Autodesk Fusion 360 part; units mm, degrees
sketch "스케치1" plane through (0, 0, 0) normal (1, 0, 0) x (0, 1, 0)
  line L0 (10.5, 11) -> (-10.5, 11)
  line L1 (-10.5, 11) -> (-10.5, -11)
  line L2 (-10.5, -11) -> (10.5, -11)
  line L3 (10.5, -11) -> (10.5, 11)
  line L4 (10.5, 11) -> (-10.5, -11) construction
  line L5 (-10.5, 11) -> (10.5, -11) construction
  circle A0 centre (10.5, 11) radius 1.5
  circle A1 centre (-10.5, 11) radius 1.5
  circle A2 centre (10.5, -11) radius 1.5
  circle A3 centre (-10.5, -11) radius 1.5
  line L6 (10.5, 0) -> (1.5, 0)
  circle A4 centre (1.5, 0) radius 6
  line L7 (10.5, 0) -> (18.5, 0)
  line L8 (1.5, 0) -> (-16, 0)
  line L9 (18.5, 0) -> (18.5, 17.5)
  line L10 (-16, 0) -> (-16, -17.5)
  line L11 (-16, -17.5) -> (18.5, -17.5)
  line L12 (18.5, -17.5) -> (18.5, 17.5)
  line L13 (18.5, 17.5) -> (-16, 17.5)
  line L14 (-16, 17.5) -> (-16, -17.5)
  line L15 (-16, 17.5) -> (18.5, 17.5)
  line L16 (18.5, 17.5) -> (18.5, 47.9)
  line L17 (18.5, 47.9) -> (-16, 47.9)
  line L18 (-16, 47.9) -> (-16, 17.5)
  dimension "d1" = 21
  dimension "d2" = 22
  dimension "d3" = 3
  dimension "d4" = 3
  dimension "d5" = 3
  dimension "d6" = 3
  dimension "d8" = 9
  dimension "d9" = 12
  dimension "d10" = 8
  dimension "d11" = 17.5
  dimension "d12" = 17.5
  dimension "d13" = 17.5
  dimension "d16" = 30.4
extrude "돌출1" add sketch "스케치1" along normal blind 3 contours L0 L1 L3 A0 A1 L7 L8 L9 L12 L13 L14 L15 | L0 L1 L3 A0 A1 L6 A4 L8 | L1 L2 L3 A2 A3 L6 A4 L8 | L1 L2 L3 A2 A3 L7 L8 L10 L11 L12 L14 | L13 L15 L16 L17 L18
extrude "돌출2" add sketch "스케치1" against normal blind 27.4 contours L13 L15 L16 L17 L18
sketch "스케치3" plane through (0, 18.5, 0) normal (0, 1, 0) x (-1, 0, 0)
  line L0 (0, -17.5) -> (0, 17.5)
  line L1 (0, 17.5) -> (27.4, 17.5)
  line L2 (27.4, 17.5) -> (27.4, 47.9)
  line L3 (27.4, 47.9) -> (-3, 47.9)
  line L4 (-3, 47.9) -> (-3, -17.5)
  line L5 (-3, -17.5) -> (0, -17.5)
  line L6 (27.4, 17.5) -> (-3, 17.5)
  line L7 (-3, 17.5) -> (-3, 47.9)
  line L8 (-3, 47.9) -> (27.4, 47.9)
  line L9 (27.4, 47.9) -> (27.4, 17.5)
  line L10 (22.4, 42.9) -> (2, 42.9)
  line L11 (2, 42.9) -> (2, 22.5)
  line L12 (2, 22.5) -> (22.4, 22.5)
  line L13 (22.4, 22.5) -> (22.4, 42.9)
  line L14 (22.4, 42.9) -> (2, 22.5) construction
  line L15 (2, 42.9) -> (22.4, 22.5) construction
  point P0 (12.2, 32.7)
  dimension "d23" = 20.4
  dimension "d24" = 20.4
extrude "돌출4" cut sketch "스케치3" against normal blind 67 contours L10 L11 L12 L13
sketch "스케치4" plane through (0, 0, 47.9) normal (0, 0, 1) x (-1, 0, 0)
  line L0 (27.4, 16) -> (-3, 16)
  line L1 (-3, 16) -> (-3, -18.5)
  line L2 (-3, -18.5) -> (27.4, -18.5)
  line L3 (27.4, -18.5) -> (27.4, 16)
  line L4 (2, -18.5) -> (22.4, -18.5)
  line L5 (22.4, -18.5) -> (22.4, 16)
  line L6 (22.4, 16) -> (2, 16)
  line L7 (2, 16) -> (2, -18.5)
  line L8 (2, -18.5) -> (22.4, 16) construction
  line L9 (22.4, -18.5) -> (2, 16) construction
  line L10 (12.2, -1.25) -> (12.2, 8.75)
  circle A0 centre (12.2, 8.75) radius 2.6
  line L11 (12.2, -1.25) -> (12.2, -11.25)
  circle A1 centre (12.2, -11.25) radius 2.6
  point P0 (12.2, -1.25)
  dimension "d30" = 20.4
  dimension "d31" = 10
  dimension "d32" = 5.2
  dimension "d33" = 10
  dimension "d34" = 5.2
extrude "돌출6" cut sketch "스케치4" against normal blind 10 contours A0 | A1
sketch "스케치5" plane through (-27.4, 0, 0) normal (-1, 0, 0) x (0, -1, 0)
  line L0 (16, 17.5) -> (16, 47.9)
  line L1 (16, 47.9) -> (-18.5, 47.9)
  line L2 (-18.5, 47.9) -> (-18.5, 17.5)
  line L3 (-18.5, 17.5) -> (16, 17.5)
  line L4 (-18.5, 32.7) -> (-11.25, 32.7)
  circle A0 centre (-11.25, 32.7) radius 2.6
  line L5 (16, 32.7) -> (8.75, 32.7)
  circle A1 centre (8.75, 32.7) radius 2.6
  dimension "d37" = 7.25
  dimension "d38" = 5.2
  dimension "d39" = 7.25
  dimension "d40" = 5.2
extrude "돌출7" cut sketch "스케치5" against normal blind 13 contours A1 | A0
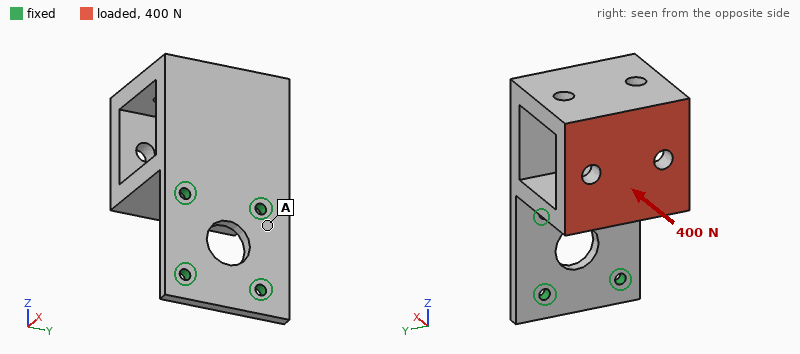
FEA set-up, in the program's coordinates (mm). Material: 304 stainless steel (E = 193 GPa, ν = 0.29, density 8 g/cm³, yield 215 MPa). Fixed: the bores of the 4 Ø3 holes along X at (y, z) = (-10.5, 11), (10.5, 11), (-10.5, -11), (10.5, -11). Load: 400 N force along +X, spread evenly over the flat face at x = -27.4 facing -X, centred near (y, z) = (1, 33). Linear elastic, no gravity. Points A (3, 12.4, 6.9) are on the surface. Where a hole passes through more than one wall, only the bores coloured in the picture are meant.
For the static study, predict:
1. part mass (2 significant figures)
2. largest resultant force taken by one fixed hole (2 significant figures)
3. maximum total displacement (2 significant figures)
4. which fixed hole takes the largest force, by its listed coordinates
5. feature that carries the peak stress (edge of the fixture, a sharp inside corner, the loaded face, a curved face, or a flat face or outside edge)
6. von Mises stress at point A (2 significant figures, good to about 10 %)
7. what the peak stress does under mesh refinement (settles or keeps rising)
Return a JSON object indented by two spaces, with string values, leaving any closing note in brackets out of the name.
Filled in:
{
  "part mass": "160 g",
  "largest resultant force taken by one fixed hole": "260 N",
  "maximum total displacement": "0.18 mm",
  "which fixed hole takes the largest force, by its listed coordinates": "(10.5, 11)",
  "feature that carries the peak stress": "edge of the fixture",
  "von Mises stress at point A": "20 MPa",
  "what the peak stress does under mesh refinement": "keeps rising"
}
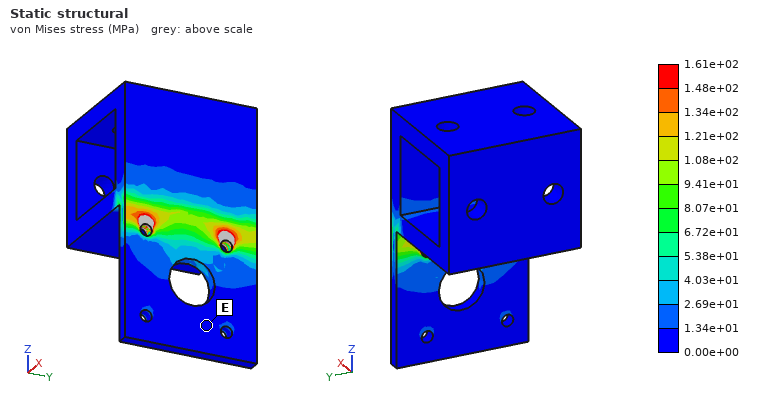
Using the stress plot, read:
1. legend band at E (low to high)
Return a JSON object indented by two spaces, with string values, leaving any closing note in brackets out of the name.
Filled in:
{
  "legend band at E": "0.00e+00 to 1.34e+01 MPa"
}
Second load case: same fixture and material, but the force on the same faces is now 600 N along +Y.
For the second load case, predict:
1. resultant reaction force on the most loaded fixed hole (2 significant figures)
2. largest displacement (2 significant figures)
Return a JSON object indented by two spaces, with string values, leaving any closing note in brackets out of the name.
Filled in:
{
  "resultant reaction force on the most loaded fixed hole": "960 N",
  "largest displacement": "37 µm"
}
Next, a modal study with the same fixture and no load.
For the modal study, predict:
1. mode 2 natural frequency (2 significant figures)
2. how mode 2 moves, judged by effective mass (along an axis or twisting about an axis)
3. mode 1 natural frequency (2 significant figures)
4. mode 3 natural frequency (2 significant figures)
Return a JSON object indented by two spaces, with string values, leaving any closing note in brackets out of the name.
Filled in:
{
  "mode 2 natural frequency": "2900 Hz",
  "how mode 2 moves, judged by effective mass": "along Y",
  "mode 1 natural frequency": "670 Hz",
  "mode 3 natural frequency": "5700 Hz"
}
